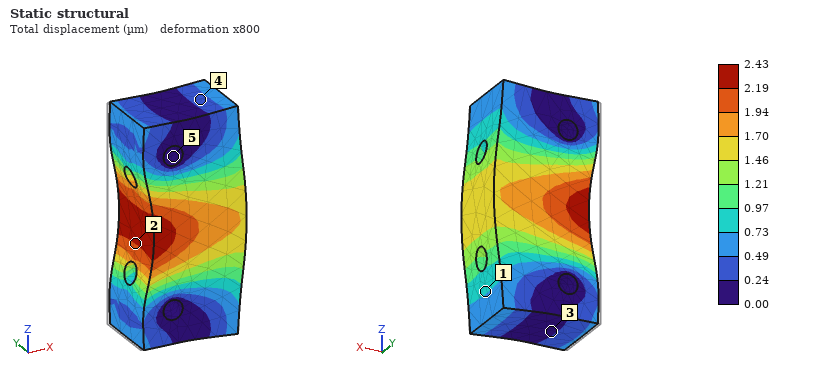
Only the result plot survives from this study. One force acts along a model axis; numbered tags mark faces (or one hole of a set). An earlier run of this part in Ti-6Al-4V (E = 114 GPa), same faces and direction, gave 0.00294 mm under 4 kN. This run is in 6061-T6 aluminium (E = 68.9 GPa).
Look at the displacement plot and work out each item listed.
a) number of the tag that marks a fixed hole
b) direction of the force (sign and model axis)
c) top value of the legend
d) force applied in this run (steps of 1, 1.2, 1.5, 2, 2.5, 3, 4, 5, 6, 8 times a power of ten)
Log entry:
5
+X
2.43 µm
2 kN
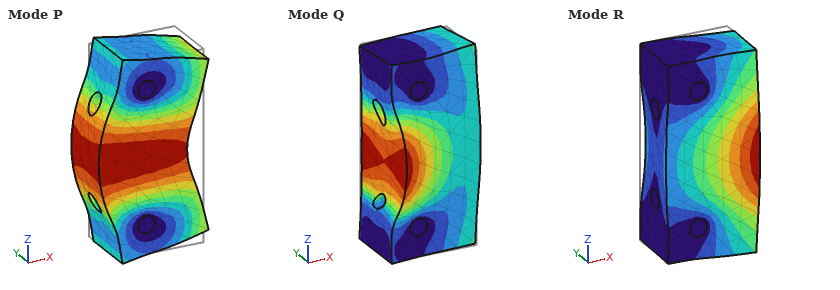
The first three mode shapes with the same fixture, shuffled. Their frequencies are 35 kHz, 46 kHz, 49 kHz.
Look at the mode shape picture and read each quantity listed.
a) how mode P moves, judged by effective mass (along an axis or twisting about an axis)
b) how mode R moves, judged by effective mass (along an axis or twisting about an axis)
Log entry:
along X
along Y
